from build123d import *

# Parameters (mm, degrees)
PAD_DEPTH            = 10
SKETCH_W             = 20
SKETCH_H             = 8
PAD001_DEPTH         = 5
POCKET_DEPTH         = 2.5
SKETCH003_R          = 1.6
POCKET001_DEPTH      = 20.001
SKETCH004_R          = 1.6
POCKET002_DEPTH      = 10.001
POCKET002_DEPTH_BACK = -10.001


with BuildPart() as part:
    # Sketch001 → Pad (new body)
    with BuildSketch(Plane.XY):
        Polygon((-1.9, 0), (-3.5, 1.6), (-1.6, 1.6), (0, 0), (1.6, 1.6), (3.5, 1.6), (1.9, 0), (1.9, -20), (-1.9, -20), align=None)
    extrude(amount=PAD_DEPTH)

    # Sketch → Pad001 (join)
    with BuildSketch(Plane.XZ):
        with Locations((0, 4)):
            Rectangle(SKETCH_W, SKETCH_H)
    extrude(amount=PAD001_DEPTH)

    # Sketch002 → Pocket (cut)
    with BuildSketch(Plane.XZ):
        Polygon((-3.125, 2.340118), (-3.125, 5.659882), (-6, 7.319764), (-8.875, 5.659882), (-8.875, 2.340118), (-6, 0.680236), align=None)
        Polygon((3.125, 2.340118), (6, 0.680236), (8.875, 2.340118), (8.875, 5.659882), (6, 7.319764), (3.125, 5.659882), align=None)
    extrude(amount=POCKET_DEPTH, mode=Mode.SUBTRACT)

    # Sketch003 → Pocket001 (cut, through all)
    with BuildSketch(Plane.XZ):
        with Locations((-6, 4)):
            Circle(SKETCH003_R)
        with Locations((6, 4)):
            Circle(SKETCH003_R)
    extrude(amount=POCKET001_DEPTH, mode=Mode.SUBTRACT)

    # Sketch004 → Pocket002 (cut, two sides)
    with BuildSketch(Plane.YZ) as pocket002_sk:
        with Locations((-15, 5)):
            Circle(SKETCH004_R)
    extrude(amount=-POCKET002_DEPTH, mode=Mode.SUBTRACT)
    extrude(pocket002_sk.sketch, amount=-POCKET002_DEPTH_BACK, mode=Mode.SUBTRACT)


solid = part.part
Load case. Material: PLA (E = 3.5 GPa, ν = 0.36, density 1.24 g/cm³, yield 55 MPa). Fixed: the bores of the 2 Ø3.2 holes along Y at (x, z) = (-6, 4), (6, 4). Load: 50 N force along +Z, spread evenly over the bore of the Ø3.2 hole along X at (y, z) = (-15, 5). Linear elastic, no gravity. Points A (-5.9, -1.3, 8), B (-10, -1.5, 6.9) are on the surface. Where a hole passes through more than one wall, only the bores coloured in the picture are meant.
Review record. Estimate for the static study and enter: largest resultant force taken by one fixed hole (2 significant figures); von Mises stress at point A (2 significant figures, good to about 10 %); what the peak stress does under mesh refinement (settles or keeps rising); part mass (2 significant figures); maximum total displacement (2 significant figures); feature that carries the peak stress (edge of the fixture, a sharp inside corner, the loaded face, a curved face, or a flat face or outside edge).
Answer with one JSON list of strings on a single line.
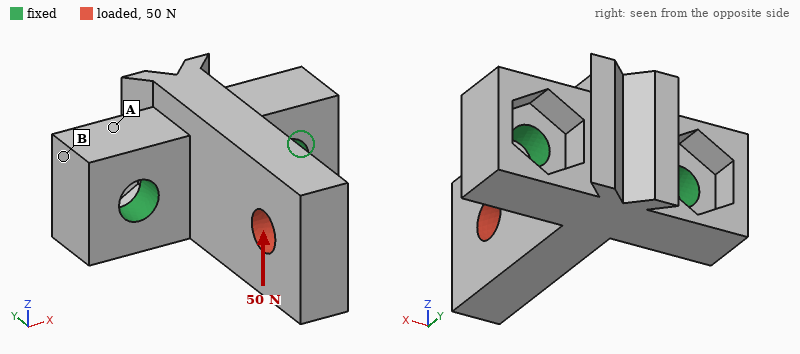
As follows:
["26 N", "7.5 MPa", "keeps rising", "1.6 g", "0.21 mm", "edge of the fixture"]
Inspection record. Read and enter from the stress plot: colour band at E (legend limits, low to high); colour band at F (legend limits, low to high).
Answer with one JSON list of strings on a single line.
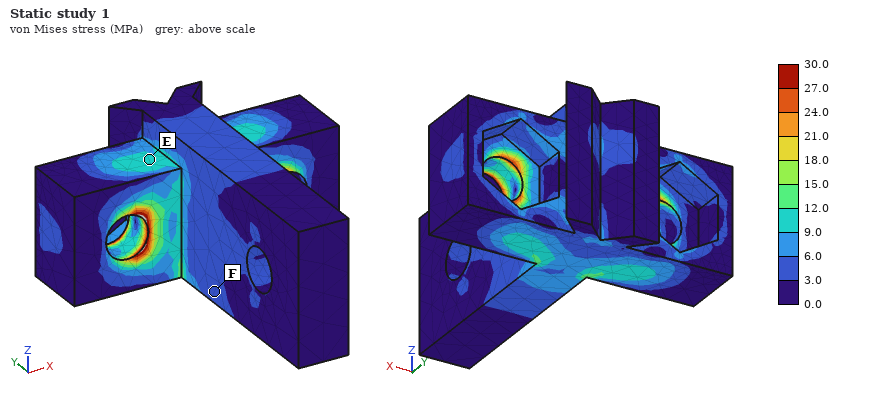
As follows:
["9.0 to 12.0 MPa", "3.0 to 6.0 MPa"]
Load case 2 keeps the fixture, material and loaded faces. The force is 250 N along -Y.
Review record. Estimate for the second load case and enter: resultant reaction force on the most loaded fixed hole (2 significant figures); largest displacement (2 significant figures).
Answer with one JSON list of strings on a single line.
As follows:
["130 N", "91 µm"]
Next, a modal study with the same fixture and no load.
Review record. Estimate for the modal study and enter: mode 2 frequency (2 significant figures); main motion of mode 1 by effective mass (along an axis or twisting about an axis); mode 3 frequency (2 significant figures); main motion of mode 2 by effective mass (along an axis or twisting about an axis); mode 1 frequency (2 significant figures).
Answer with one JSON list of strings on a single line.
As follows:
["4100 Hz", "along X", "10 kHz", "along Z", "3700 Hz"]
